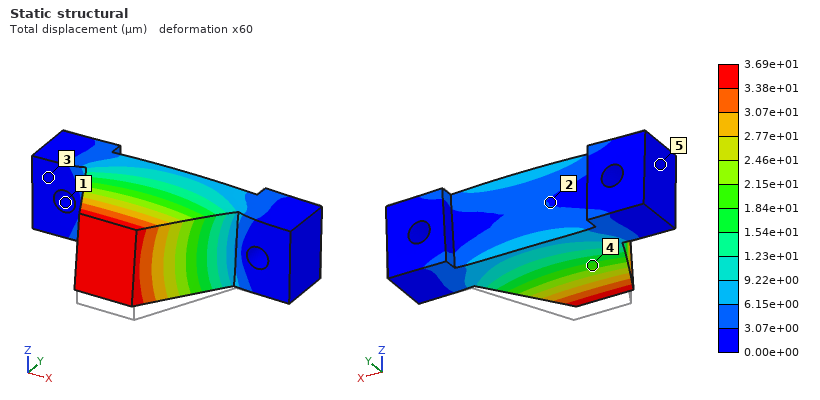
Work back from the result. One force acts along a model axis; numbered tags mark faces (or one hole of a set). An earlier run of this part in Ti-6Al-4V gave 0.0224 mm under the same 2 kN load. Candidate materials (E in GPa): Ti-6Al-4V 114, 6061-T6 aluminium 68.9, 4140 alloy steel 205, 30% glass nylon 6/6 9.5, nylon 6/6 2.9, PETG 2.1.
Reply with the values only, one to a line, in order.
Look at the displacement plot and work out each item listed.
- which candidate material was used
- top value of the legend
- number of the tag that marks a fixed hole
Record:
6061-T6 aluminium
3.69e+01 µm
1
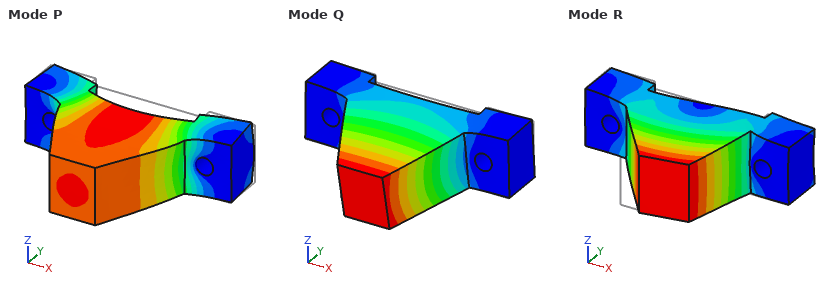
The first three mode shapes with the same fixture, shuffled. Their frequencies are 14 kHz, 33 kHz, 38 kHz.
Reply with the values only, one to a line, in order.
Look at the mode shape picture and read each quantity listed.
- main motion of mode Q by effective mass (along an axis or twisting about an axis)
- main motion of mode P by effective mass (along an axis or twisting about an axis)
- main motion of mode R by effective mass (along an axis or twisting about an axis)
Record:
along Z
along Y
along X
